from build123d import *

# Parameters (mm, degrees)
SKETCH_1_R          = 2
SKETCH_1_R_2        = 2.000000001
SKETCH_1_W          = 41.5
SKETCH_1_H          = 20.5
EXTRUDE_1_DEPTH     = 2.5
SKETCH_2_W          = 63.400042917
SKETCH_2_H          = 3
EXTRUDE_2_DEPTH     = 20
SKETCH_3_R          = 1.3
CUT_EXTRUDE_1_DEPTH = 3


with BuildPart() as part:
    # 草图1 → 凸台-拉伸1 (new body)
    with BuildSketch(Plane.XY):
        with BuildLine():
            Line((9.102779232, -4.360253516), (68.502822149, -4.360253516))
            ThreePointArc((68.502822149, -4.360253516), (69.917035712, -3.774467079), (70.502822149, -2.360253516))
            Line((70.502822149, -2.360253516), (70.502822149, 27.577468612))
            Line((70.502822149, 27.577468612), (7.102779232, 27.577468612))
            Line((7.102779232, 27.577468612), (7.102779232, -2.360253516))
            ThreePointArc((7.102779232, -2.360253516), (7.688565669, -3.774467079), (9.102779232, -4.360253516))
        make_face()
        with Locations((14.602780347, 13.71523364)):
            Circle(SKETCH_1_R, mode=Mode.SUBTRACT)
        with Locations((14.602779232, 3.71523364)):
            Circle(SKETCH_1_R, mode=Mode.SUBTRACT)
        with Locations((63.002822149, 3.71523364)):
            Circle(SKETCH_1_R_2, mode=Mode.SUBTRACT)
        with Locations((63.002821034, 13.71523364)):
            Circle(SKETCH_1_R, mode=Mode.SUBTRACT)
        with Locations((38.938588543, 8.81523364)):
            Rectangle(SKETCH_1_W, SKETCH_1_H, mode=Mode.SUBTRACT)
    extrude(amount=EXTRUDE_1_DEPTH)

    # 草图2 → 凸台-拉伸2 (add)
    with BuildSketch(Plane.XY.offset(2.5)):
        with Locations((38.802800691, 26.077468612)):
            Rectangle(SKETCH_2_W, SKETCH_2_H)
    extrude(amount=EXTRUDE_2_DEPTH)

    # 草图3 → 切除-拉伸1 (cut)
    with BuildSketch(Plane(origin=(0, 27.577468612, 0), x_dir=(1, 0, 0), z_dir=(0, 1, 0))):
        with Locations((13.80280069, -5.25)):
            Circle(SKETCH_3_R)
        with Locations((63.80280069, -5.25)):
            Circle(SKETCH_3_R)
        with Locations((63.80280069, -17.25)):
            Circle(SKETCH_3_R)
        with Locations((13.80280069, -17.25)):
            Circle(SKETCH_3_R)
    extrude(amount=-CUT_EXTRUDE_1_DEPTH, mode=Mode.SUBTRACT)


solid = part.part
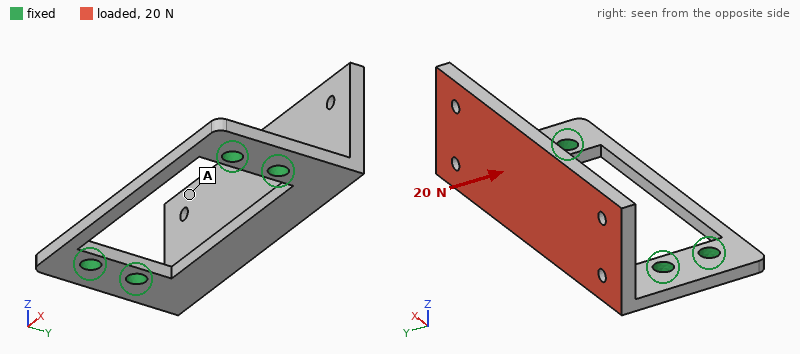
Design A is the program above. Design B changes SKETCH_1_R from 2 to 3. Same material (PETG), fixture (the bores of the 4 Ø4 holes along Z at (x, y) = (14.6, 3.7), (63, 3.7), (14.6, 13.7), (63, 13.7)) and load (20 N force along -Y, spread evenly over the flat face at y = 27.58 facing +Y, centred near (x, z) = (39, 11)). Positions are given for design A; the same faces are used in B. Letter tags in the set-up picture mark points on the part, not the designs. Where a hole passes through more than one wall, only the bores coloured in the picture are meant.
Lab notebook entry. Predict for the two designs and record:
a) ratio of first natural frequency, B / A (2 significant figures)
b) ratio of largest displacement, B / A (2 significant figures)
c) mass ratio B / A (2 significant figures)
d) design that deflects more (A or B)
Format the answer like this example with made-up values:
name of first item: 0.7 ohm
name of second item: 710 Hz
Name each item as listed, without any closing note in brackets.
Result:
ratio of first natural frequency, B / A: 1.1
ratio of largest displacement, B / A: 0.88
mass ratio B / A: 0.98
design that deflects more: A
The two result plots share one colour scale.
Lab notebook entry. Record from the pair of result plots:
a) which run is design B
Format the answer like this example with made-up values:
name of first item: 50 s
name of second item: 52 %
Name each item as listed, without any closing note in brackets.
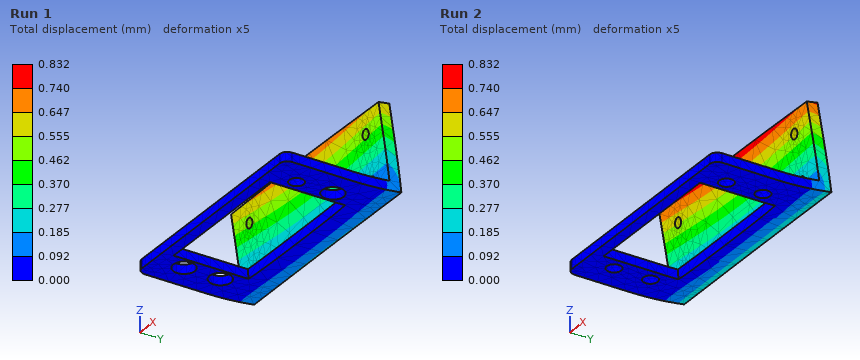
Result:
which run is design B: Run 1
